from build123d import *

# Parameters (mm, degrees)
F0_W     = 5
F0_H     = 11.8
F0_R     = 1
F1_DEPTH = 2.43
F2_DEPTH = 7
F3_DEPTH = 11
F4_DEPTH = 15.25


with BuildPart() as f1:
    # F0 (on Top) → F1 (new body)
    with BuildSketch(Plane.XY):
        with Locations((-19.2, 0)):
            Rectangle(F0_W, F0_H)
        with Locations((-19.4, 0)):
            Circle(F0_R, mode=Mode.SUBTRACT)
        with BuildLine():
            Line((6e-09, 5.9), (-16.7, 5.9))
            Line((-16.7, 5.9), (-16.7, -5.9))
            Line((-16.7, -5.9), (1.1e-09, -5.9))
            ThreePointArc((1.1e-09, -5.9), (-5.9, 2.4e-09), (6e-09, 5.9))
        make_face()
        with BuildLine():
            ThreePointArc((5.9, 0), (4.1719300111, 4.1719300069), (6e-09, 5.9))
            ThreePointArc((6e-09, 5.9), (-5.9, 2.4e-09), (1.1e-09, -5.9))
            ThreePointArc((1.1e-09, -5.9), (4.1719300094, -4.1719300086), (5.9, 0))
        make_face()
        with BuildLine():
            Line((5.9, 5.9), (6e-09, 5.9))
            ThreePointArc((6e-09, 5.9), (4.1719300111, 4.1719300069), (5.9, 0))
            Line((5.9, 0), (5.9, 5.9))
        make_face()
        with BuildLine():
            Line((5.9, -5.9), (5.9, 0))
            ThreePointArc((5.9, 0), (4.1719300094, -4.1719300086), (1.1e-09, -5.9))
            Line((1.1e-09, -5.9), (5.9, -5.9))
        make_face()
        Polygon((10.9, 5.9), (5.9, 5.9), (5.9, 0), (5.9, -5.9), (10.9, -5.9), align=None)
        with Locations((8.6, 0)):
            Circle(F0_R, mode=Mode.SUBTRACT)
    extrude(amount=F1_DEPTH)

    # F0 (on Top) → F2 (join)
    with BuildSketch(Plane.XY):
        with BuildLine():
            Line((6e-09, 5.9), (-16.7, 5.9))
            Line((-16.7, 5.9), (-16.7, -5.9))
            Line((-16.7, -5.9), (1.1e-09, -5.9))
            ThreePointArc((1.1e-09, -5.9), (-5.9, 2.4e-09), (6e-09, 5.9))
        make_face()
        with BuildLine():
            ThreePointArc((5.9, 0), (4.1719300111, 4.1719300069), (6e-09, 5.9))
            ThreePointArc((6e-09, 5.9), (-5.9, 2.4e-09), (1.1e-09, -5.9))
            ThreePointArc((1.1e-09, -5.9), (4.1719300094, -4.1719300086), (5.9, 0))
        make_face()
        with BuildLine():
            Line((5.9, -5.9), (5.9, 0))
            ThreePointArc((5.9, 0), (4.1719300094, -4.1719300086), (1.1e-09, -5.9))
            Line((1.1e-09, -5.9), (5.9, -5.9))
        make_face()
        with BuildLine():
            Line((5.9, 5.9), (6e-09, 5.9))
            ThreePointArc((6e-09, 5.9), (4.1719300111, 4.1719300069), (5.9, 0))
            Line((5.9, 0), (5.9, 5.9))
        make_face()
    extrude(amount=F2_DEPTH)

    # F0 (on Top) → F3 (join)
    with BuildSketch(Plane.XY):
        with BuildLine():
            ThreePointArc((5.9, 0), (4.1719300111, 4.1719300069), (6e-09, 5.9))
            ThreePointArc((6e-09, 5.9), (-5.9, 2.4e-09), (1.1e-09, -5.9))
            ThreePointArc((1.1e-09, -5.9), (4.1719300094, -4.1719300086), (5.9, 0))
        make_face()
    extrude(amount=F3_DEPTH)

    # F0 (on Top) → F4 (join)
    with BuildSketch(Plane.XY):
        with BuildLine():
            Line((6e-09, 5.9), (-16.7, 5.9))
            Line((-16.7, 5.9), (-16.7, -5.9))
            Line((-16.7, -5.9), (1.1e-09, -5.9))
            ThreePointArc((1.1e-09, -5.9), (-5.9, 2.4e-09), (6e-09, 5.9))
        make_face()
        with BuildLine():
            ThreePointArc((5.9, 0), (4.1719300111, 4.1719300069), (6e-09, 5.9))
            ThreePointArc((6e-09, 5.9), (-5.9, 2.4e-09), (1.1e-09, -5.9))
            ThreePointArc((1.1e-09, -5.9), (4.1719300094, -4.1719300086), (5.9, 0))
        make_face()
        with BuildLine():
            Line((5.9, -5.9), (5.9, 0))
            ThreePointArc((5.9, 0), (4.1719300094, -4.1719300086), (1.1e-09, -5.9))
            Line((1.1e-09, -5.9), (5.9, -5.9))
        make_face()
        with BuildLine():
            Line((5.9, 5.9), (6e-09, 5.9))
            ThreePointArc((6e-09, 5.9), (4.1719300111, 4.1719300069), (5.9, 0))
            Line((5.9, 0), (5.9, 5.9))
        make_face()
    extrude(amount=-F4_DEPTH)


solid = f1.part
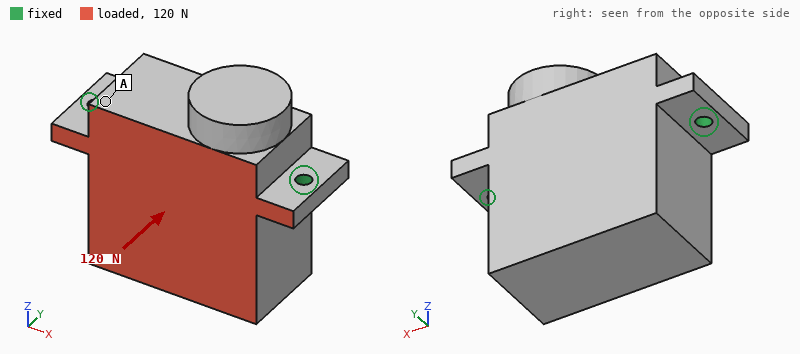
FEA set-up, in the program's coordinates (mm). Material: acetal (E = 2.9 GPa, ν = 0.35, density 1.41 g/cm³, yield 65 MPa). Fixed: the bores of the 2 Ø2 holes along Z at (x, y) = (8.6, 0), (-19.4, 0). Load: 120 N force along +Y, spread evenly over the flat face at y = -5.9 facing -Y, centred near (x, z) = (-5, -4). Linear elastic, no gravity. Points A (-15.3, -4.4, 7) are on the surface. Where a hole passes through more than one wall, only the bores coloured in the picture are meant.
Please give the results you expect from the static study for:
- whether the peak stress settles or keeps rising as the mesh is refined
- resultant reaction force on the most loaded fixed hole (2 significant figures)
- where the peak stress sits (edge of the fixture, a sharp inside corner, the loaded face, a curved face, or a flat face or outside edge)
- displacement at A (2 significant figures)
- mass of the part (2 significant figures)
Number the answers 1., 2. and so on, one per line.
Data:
1. keeps rising
2. 60 N
3. edge of the fixture
4. 0.11 mm
5. 9.4 g
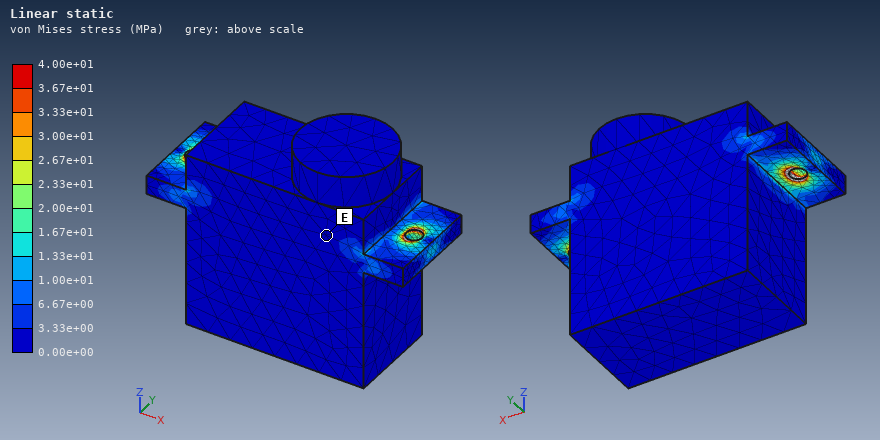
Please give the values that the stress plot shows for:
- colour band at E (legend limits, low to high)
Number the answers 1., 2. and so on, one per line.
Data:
1. 0.00e+00 to 3.33e+00 MPa
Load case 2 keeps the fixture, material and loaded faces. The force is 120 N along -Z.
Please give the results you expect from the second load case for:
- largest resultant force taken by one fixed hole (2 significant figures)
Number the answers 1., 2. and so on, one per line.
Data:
1. 60 N
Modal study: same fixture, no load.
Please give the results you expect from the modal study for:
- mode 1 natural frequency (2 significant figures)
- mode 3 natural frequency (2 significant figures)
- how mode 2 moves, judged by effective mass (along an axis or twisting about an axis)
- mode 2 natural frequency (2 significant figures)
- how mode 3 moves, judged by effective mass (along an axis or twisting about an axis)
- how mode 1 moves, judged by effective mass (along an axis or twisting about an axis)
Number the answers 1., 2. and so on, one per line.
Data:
1. 1100 Hz
2. 4600 Hz
3. along Z
4. 4100 Hz
5. along X
6. along Y
